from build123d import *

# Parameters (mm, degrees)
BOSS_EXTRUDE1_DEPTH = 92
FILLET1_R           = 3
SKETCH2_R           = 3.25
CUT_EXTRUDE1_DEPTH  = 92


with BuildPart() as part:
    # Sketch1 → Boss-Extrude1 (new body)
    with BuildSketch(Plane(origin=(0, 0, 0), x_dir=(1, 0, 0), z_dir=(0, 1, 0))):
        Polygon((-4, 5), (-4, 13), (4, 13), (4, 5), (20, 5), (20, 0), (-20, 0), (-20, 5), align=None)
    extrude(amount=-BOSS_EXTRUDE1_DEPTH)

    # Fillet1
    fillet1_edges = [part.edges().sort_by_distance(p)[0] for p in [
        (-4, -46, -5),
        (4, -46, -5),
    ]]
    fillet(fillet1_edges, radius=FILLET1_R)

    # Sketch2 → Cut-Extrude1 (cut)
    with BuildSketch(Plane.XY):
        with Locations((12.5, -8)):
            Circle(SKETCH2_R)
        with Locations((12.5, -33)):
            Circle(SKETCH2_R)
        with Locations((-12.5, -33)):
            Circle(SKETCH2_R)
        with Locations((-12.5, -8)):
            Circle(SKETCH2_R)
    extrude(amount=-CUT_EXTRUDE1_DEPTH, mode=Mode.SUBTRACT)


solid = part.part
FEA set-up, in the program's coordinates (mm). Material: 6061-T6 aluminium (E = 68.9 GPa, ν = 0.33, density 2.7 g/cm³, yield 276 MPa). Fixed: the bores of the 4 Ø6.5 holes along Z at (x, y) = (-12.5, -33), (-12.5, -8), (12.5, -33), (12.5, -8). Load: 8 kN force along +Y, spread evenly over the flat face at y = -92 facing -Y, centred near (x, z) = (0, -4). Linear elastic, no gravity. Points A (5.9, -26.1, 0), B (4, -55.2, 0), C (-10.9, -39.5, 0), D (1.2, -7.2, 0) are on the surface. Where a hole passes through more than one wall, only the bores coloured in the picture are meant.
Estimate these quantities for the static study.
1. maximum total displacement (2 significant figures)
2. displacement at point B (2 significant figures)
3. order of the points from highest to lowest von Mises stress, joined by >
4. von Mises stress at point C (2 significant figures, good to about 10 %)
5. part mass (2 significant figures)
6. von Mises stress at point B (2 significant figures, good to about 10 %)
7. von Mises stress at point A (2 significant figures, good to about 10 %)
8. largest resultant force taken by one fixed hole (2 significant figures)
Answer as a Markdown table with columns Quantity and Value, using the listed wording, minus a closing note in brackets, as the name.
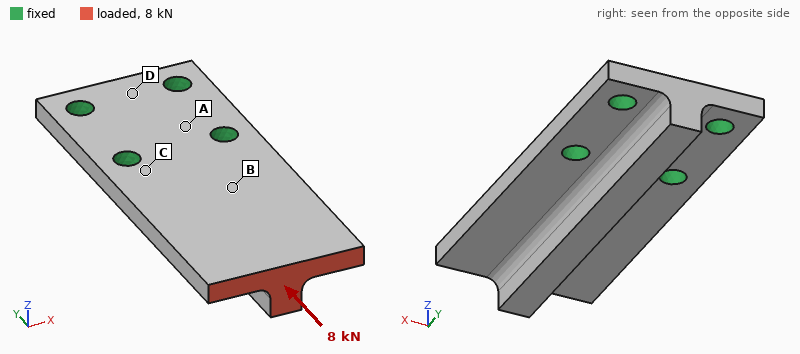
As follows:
| Quantity | Value |
|---|---|
| maximum total displacement | 53 µm |
| displacement at point B | 15 µm |
| order of the points from highest to lowest von Mises stress, joined by > | C > B > A > D |
| von Mises stress at point C | 37 MPa |
| part mass | 65 g |
| von Mises stress at point B | 27 MPa |
| von Mises stress at point A | 12 MPa |
| largest resultant force taken by one fixed hole | 3.4 kN |
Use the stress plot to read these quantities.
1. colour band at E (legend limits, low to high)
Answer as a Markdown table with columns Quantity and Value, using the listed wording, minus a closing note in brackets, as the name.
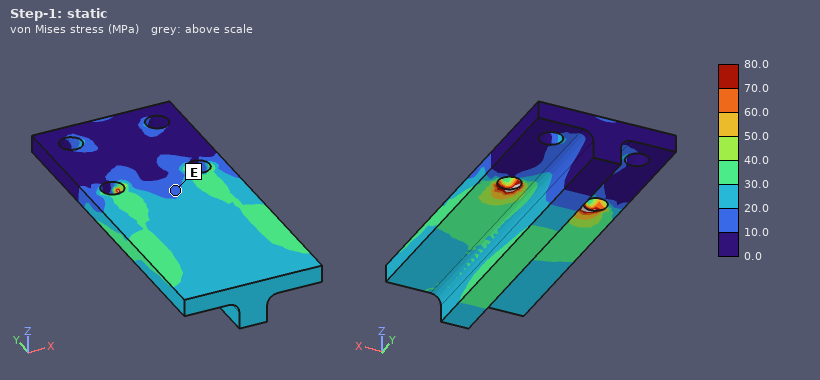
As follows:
| Quantity | Value |
|---|---|
| colour band at E | 10.0 to 20.0 MPa |
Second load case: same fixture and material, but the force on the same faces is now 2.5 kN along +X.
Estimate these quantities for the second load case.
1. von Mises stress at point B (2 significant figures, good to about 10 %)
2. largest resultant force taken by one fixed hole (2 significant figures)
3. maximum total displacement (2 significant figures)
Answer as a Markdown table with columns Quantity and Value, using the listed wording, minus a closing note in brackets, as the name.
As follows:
| Quantity | Value |
|---|---|
| von Mises stress at point B | 27 MPa |
| largest resultant force taken by one fixed hole | 5.0 kN |
| maximum total displacement | 0.13 mm |
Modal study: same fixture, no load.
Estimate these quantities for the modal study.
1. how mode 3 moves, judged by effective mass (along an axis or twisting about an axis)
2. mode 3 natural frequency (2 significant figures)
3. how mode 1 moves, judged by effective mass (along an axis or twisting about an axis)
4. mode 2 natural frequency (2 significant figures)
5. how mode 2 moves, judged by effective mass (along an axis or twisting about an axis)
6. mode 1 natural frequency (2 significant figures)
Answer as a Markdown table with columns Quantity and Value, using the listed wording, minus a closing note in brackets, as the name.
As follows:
| Quantity | Value |
|---|---|
| how mode 3 moves, judged by effective mass | along X |
| mode 3 natural frequency | 6600 Hz |
| how mode 1 moves, judged by effective mass | along Z |
| mode 2 natural frequency | 5000 Hz |
| how mode 2 moves, judged by effective mass | twisting about Y |
| mode 1 natural frequency | 2100 Hz |
